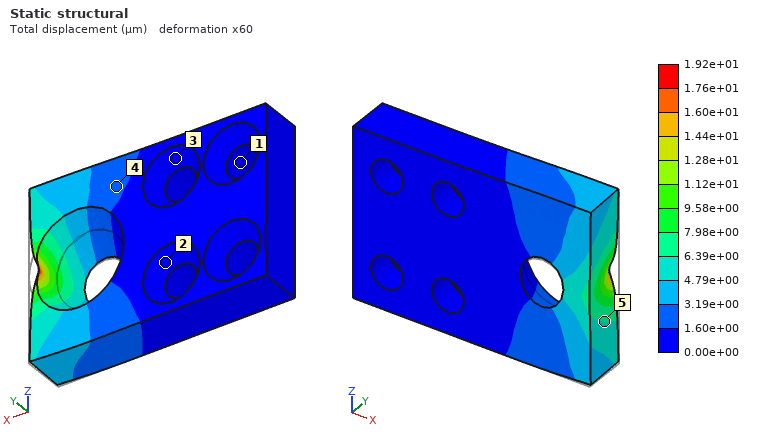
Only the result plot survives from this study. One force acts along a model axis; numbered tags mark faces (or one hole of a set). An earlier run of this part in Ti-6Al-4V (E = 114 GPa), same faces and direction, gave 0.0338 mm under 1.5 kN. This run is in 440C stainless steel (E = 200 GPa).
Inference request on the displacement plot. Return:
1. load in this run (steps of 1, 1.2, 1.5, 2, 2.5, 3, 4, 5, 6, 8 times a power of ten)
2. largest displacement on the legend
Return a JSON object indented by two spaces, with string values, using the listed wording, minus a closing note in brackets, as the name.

{
  "load in this run": "1.5 kN",
  "largest displacement on the legend": "1.92e+01 µm"
}
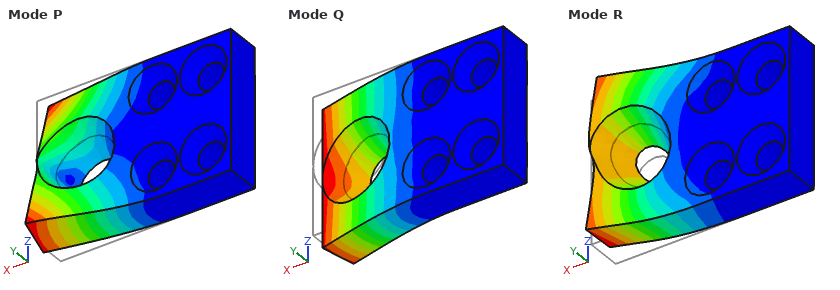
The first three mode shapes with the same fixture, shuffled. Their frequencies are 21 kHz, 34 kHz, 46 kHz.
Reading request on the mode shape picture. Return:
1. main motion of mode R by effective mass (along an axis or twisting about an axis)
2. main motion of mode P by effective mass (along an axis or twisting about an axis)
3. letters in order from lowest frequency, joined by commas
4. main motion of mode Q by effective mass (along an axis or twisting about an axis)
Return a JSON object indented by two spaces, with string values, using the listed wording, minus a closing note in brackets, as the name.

{
  "main motion of mode R by effective mass": "along Z",
  "main motion of mode P by effective mass": "twisting about X",
  "letters in order from lowest frequency, joined by commas": "Q, P, R",
  "main motion of mode Q by effective mass": "along Y"
}
